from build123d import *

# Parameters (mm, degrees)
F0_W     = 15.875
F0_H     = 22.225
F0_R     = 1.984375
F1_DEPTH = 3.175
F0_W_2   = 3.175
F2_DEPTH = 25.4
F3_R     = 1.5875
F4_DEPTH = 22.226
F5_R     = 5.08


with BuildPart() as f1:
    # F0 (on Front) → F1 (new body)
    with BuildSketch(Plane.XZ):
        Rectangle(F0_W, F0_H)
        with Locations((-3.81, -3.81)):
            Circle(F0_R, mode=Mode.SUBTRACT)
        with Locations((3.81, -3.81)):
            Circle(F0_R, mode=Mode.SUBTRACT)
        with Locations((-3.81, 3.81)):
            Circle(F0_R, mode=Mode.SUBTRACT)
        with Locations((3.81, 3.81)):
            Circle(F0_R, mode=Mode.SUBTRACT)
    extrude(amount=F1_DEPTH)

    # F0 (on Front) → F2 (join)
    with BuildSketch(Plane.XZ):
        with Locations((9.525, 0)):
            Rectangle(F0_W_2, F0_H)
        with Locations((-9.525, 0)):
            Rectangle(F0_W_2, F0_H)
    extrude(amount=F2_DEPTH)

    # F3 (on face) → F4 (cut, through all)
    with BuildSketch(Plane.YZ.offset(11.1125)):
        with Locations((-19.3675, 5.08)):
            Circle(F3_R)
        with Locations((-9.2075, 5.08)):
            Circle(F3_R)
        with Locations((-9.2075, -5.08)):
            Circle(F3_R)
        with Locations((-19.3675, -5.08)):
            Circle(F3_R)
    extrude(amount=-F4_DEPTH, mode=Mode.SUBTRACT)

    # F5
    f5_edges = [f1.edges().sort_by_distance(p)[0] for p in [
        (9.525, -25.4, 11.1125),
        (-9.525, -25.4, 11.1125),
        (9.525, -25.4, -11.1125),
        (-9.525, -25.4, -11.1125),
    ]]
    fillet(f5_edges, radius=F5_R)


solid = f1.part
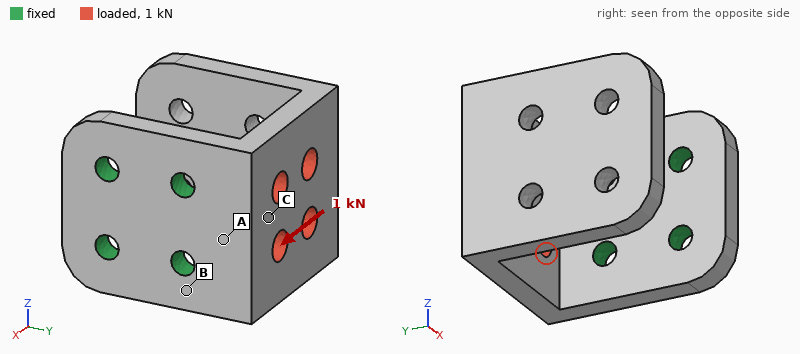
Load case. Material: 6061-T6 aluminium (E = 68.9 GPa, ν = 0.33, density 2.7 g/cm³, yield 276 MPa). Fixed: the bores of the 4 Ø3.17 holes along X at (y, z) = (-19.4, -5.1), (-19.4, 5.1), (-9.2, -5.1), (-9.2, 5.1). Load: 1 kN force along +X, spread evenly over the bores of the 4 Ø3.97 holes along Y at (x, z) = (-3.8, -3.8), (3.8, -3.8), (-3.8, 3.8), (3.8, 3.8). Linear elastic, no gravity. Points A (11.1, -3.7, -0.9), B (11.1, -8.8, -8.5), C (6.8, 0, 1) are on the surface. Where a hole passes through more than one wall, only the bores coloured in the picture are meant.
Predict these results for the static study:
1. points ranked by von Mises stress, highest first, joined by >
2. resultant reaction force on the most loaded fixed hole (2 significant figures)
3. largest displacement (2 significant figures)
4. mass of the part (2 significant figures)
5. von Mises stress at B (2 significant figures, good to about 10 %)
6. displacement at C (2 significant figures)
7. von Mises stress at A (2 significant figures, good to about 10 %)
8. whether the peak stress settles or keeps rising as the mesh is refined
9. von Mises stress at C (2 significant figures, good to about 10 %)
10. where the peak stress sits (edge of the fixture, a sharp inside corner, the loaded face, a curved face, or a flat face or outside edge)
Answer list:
B > A > C
560 N
0.17 mm
12 g
77 MPa
0.046 mm
49 MPa
keeps rising
22 MPa
edge of the fixture
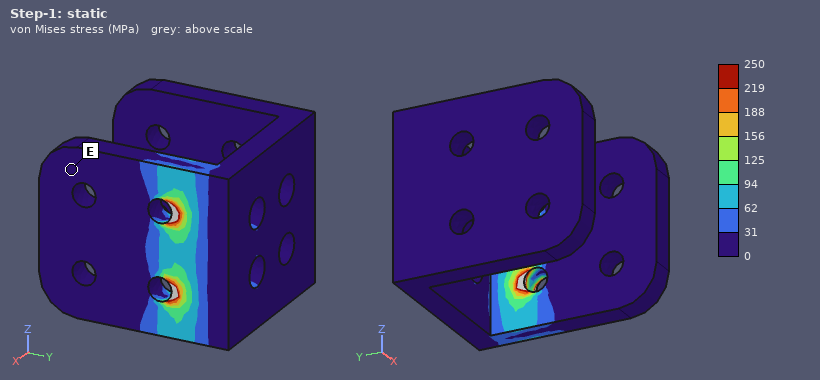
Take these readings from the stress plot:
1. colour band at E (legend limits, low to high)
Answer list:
0 to 31 MPa
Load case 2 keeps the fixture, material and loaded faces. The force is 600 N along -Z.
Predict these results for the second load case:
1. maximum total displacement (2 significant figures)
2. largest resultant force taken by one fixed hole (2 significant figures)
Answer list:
96 µm
590 N
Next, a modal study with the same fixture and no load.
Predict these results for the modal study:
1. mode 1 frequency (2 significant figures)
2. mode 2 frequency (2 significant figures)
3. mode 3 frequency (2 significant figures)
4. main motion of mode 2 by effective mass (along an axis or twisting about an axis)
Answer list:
1500 Hz
2500 Hz
4100 Hz
along Z
